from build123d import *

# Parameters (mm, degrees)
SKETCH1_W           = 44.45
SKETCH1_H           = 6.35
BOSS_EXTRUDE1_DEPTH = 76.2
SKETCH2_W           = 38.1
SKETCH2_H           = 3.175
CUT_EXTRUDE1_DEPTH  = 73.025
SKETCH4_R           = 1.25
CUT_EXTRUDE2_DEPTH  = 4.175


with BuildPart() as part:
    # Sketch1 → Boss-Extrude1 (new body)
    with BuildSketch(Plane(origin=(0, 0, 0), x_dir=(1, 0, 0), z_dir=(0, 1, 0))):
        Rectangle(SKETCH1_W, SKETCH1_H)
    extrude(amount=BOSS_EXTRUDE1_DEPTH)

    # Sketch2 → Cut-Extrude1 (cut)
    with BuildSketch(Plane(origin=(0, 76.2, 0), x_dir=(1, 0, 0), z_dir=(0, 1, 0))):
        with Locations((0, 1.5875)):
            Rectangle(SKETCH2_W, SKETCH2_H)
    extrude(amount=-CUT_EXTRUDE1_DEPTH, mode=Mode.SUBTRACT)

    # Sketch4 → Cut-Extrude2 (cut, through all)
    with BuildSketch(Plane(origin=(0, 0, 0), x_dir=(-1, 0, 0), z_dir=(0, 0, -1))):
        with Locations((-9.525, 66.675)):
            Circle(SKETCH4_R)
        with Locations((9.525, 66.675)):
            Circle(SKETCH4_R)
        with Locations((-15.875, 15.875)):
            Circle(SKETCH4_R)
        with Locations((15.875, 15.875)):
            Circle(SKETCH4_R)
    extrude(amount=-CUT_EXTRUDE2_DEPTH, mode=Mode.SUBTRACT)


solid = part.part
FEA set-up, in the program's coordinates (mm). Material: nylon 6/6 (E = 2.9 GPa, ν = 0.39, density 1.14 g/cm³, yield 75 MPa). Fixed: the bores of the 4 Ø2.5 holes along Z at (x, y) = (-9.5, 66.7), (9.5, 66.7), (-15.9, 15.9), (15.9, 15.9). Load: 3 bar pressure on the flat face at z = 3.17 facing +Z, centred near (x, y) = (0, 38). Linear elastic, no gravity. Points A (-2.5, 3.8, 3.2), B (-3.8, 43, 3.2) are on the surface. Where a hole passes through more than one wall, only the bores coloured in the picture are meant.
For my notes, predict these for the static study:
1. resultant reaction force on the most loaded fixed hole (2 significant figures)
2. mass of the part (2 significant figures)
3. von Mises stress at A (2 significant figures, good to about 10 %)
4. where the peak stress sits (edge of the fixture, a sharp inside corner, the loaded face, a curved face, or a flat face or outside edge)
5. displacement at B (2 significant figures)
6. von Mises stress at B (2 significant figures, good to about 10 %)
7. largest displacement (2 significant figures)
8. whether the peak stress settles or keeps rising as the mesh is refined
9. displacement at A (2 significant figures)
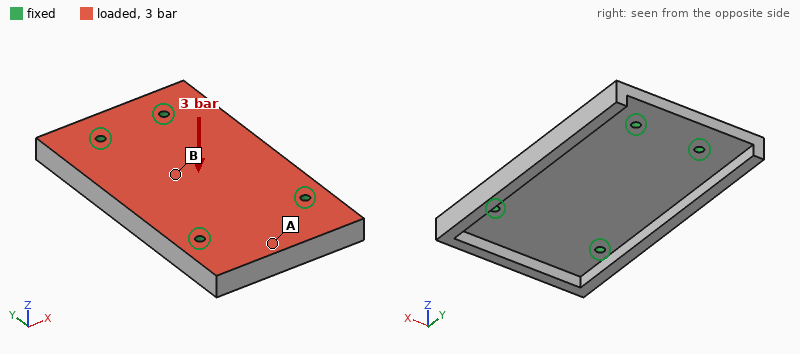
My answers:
280 N
14 g
6.8 MPa
edge of the fixture
0.57 mm
13 MPa
0.59 mm
keeps rising
0.14 mm
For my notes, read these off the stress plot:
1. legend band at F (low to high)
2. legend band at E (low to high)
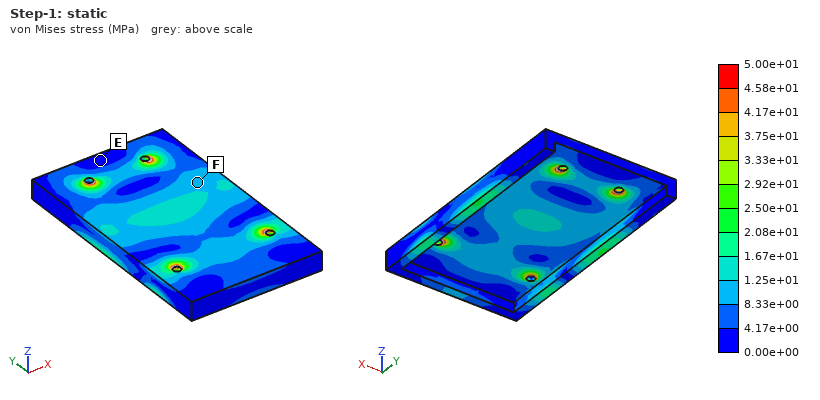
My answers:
8.33e+00 to 1.25e+01 MPa
0.00e+00 to 4.17e+00 MPa
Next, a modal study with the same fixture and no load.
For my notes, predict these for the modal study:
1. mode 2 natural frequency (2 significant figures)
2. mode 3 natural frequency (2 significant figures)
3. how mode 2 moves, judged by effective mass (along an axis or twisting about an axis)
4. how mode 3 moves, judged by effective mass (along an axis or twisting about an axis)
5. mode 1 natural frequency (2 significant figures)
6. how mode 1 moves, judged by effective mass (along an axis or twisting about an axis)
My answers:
2300 Hz
2600 Hz
twisting about Y
along Z
1900 Hz
along Z
